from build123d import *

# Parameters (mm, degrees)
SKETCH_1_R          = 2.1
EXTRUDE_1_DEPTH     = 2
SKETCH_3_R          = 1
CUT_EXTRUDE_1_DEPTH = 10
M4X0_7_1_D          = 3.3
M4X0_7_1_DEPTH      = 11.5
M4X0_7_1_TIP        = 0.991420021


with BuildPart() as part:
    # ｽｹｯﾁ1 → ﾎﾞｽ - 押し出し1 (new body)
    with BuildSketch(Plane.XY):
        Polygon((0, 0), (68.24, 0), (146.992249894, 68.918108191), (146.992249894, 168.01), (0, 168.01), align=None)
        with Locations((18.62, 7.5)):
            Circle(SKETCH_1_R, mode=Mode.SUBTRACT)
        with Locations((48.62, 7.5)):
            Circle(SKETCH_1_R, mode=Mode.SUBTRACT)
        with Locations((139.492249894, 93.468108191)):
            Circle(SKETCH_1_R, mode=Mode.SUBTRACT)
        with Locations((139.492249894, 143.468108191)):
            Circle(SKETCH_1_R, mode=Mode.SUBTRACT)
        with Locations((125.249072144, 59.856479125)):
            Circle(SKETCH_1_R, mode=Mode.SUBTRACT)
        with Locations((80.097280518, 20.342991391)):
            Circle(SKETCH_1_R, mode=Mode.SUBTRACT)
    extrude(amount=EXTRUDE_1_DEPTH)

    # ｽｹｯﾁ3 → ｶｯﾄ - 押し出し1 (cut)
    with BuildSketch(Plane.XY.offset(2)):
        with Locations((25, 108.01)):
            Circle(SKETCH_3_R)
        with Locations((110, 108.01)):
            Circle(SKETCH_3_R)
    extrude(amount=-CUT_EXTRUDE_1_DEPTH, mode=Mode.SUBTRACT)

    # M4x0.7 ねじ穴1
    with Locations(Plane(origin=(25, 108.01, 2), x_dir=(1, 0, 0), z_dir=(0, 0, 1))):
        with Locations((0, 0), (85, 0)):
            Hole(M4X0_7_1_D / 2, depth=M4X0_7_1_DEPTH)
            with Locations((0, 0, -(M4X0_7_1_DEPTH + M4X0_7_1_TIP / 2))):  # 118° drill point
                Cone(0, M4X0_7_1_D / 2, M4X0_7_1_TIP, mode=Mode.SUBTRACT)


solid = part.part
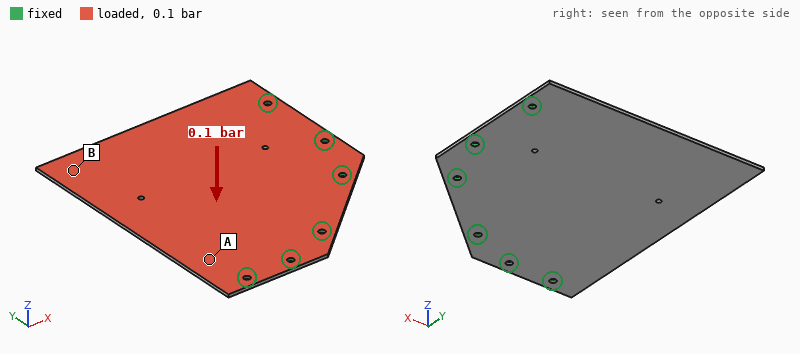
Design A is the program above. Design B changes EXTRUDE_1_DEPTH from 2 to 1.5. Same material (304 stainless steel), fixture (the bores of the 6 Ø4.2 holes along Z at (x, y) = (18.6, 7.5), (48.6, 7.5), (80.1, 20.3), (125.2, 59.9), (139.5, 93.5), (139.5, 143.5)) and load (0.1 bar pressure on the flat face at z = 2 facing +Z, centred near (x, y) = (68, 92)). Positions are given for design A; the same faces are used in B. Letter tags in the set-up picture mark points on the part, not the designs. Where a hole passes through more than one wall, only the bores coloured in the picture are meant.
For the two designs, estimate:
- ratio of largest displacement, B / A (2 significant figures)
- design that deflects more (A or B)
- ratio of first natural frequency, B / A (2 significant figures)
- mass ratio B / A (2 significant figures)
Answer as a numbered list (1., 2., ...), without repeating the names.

1. 2.4
2. B
3. 0.75
4. 0.75
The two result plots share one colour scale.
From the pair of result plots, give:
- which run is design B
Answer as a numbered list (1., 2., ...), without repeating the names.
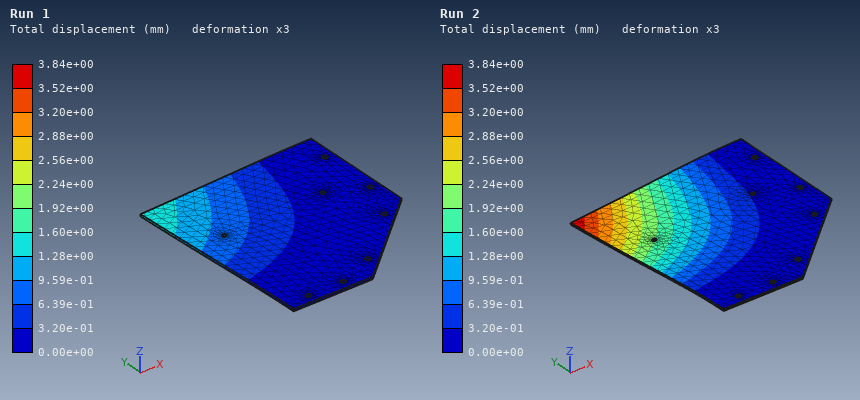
1. Run 2
